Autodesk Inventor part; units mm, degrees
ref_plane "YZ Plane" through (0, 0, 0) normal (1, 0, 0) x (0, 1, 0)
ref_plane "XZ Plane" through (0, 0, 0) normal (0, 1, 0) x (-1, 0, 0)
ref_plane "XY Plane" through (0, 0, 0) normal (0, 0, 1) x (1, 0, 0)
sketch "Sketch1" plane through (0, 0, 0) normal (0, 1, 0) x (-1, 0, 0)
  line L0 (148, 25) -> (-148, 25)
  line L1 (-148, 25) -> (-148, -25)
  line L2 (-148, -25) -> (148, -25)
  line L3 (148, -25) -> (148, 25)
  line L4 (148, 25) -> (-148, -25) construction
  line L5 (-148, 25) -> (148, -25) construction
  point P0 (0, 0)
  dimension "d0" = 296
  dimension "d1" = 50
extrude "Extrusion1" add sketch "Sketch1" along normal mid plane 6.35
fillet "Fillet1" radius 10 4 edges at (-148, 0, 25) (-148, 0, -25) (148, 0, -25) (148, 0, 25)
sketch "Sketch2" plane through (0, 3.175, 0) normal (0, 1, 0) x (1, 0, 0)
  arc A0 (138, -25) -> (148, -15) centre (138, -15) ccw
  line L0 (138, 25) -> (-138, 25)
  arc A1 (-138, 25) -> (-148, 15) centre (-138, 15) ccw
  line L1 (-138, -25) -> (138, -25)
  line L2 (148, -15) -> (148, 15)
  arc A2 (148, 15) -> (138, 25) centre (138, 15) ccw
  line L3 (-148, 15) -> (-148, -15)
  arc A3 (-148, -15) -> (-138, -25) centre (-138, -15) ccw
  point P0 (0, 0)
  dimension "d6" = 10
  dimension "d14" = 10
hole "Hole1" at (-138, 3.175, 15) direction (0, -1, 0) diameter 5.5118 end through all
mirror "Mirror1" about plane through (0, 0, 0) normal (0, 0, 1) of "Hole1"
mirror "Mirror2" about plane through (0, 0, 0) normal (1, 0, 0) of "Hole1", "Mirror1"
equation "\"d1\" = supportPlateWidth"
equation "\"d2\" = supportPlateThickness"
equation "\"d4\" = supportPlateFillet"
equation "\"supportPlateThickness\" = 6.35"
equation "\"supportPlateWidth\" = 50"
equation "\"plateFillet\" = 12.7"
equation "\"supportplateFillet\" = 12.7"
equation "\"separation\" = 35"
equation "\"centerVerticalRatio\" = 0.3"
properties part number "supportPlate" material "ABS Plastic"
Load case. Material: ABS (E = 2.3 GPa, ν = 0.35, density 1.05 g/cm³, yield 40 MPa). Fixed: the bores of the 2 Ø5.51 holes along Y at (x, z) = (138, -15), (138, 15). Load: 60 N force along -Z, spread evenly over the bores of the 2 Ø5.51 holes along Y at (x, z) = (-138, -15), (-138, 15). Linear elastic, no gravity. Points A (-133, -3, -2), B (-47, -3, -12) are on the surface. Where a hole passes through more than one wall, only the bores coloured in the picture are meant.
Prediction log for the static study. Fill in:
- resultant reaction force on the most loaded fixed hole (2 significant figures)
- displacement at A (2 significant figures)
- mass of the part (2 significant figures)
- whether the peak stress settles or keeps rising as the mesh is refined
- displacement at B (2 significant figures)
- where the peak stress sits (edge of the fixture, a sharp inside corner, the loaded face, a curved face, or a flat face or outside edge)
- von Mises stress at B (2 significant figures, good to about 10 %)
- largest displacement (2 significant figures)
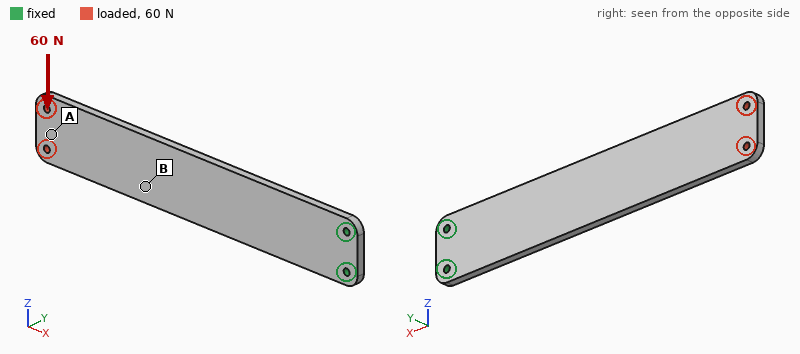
510 N
2.9 mm
97 g
keeps rising
1.6 mm
edge of the fixture
1.1 MPa
3.1 mm
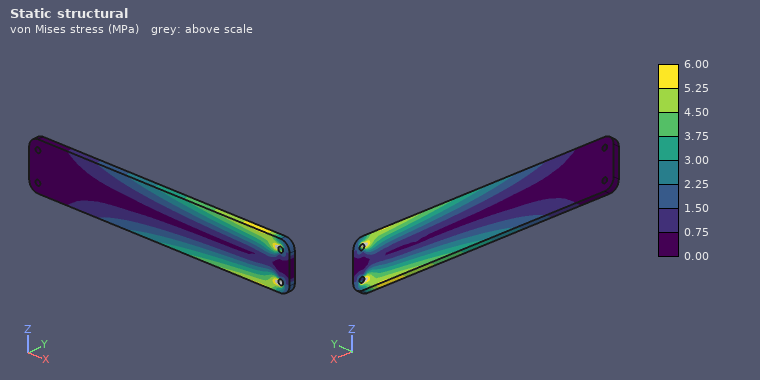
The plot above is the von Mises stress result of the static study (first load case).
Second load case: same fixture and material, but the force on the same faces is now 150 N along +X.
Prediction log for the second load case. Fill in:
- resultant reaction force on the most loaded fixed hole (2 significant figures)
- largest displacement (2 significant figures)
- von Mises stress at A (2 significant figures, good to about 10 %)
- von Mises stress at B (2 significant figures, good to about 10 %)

76 N
61 µm
0.25 MPa
0.47 MPa
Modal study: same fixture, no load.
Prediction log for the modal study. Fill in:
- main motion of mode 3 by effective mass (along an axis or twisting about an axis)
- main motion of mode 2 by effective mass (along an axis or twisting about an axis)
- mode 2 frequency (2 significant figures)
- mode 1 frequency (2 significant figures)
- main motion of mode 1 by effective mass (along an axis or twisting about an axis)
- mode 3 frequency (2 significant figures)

along Z
along Y
120 Hz
19 Hz
along Y
140 Hz
